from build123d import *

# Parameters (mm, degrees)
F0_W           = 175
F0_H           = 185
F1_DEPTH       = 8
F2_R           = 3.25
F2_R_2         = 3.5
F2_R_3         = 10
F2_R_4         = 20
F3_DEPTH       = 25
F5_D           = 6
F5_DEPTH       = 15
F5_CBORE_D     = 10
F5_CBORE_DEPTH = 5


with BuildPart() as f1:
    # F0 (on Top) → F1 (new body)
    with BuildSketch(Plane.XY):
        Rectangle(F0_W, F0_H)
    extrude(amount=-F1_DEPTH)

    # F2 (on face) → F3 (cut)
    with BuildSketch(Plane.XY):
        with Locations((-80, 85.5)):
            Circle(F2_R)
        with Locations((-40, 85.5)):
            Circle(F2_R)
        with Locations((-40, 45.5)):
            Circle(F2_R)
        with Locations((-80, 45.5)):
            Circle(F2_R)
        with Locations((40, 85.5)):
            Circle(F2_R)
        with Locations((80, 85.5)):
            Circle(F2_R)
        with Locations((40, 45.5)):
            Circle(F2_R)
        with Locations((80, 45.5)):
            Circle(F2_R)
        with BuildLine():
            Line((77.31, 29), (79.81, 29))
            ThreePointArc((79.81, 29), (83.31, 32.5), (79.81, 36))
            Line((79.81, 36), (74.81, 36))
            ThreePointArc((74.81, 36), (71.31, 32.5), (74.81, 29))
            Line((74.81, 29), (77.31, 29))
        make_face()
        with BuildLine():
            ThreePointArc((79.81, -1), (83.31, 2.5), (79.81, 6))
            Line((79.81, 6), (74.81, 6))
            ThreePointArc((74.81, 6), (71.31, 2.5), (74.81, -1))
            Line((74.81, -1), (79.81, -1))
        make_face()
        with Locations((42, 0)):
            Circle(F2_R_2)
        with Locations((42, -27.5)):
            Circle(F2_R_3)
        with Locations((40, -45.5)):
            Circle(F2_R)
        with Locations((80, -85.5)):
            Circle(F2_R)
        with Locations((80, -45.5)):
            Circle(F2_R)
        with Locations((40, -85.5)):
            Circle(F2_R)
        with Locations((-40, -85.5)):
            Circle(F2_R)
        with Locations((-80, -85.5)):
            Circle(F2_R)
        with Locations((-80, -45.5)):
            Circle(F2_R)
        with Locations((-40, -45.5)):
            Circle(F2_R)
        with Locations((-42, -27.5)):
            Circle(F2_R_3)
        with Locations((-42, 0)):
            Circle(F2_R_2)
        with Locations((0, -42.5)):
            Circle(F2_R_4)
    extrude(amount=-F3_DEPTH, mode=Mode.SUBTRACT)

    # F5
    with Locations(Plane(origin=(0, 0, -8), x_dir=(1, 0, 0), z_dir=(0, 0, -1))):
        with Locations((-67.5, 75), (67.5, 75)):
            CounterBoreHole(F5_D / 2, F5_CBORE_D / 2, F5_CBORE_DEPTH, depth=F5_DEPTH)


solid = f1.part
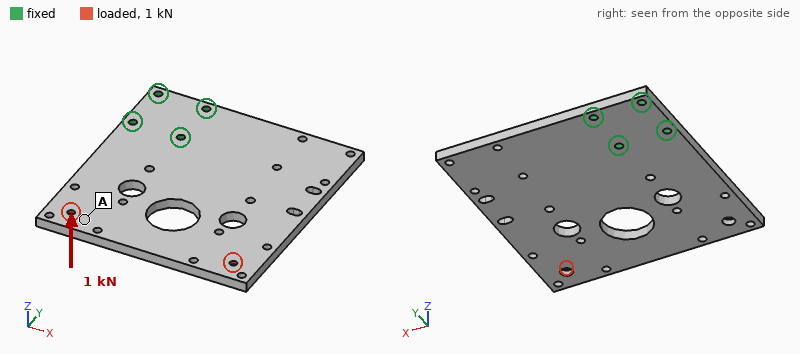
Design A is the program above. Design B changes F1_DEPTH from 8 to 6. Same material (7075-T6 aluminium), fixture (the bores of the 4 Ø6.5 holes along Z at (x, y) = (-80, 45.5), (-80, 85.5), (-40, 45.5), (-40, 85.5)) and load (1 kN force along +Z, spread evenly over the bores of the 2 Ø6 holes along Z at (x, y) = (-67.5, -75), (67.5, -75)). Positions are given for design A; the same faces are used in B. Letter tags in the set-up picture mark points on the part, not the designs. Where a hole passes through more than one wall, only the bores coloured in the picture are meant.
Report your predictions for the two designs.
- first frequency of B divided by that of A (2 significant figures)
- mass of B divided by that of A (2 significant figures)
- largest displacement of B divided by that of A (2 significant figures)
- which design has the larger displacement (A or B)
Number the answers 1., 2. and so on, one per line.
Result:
1. 0.76
2. 0.75
3. 2.3
4. B
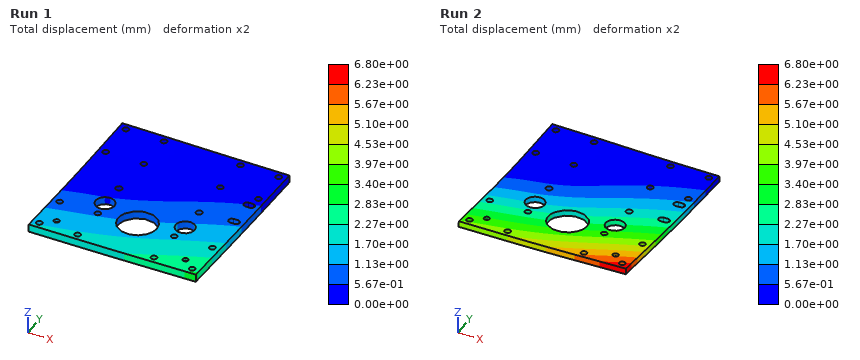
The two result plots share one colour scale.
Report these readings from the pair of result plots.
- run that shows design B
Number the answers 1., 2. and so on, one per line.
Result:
1. Run 2
